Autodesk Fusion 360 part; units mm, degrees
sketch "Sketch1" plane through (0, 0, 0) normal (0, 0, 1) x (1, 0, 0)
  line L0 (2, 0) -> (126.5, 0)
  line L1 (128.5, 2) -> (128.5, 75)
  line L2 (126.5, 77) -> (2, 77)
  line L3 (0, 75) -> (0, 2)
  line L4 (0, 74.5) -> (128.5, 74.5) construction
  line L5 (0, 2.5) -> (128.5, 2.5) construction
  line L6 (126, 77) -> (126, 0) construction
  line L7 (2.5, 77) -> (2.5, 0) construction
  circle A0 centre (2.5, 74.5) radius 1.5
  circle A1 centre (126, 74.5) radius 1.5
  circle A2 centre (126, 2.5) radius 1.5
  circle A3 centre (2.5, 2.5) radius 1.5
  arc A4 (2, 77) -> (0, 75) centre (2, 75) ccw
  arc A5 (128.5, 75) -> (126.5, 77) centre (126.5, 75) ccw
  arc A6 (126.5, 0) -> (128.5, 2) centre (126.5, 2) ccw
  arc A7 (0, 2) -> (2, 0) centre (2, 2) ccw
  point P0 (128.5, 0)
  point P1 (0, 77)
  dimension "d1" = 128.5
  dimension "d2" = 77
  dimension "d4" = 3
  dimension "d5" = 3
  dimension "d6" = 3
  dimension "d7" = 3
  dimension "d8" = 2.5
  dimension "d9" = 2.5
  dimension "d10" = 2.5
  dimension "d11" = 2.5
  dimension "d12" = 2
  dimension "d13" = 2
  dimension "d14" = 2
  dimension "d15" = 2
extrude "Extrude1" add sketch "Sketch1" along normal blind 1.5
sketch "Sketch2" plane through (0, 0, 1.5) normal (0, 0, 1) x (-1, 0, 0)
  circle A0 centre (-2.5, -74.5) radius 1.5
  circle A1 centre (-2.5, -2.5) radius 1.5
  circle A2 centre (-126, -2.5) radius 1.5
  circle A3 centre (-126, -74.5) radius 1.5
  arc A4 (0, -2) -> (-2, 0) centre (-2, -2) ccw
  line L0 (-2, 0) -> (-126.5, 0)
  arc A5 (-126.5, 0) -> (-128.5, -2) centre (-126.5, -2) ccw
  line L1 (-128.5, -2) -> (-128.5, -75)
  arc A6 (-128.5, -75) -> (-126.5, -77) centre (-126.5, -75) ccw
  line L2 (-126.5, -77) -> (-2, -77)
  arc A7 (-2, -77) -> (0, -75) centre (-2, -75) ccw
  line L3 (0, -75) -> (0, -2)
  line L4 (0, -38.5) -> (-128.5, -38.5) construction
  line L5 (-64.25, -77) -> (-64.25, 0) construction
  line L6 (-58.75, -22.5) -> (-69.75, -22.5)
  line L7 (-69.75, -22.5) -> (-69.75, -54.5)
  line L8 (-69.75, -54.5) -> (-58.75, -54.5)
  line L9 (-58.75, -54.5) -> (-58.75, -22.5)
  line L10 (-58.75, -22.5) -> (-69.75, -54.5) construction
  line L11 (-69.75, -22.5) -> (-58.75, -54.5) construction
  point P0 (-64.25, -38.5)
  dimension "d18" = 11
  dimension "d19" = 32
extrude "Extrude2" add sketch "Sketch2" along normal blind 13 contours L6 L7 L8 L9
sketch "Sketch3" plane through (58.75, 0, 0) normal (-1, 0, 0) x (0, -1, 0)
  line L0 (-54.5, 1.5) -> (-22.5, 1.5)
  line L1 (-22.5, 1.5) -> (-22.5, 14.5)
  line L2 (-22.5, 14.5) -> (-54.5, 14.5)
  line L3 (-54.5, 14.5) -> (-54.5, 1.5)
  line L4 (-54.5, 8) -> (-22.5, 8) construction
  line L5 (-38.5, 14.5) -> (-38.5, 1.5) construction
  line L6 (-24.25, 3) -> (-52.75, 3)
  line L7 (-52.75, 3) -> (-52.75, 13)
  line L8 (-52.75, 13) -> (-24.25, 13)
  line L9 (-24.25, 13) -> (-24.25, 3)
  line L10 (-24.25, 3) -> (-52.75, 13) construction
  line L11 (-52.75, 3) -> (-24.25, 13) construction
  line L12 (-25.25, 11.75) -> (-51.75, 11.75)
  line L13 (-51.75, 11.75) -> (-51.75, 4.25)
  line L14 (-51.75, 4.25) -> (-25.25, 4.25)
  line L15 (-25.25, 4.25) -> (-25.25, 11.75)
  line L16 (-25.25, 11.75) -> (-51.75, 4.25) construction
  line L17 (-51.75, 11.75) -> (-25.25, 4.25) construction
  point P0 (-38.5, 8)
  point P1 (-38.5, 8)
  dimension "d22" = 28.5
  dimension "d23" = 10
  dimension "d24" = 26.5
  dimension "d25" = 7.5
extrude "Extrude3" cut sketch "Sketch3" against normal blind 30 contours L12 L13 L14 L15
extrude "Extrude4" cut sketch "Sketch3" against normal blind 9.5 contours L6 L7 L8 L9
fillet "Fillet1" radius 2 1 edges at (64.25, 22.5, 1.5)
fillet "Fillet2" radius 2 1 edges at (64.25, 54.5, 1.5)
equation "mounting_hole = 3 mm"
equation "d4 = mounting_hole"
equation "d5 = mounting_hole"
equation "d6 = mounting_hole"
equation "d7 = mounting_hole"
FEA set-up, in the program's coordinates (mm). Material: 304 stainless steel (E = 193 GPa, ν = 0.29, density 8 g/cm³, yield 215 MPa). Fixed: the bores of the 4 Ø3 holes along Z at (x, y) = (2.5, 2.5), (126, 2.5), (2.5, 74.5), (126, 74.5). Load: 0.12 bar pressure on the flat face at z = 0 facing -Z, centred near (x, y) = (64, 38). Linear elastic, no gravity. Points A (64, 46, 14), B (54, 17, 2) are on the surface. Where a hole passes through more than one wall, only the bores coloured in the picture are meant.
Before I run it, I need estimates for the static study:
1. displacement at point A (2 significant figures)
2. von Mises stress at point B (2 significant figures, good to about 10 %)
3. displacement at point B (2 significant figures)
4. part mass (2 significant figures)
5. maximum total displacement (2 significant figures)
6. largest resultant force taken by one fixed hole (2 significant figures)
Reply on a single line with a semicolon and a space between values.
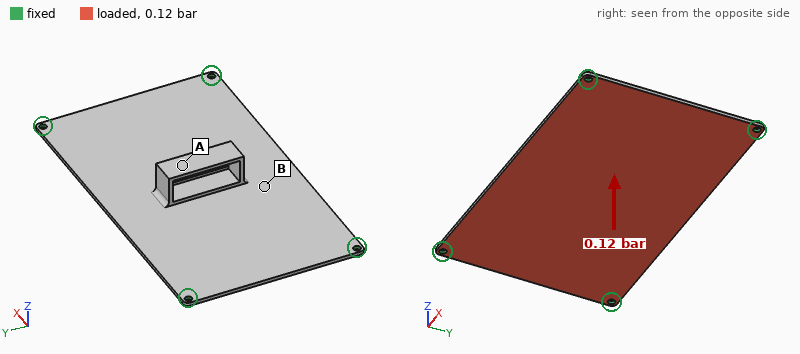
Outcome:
0.21 mm; 25 MPa; 0.21 mm; 130 g; 0.21 mm; 30 N
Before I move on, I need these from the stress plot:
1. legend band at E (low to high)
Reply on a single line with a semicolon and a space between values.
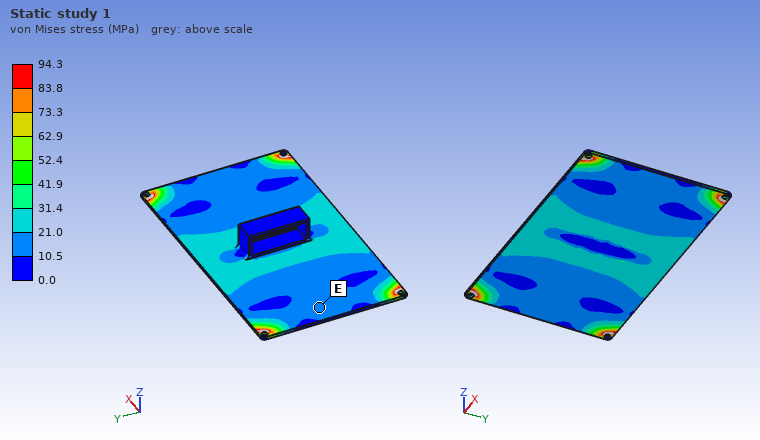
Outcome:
10.5 to 21.0 MPa
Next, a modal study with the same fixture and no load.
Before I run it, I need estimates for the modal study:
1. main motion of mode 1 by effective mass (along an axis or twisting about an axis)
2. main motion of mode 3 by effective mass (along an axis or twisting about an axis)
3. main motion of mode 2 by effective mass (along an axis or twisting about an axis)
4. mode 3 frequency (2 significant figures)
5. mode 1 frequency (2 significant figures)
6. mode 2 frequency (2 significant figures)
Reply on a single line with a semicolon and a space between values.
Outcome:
along Z; twisting about Y; twisting about X; 990 Hz; 350 Hz; 670 Hz
